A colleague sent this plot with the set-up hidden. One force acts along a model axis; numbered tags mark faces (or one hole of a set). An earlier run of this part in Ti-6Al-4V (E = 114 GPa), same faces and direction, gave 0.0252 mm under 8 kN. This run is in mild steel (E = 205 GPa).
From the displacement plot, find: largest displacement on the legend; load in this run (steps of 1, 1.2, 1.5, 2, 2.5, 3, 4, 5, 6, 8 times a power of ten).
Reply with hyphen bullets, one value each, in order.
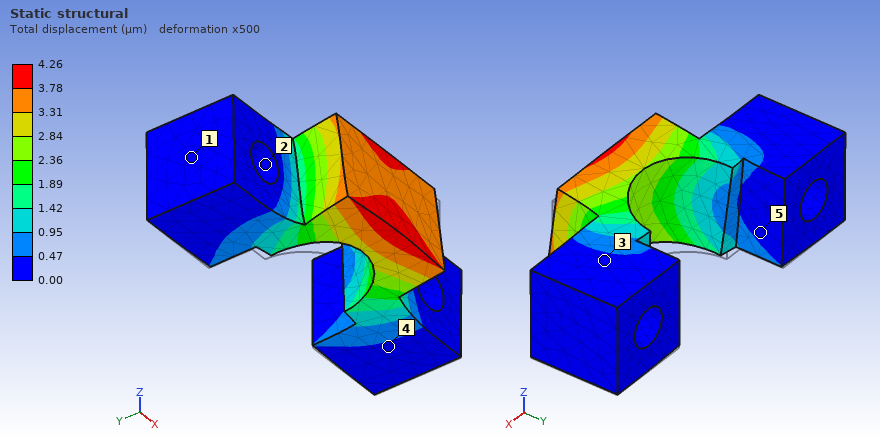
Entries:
- 4.26 µm
- 2.5 kN
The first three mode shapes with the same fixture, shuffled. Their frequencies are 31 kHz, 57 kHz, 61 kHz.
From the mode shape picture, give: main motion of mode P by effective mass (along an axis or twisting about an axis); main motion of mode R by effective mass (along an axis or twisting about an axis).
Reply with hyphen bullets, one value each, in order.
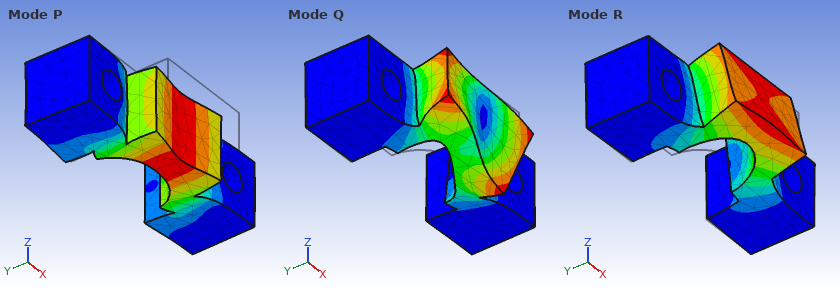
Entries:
- along Y
- along Z
